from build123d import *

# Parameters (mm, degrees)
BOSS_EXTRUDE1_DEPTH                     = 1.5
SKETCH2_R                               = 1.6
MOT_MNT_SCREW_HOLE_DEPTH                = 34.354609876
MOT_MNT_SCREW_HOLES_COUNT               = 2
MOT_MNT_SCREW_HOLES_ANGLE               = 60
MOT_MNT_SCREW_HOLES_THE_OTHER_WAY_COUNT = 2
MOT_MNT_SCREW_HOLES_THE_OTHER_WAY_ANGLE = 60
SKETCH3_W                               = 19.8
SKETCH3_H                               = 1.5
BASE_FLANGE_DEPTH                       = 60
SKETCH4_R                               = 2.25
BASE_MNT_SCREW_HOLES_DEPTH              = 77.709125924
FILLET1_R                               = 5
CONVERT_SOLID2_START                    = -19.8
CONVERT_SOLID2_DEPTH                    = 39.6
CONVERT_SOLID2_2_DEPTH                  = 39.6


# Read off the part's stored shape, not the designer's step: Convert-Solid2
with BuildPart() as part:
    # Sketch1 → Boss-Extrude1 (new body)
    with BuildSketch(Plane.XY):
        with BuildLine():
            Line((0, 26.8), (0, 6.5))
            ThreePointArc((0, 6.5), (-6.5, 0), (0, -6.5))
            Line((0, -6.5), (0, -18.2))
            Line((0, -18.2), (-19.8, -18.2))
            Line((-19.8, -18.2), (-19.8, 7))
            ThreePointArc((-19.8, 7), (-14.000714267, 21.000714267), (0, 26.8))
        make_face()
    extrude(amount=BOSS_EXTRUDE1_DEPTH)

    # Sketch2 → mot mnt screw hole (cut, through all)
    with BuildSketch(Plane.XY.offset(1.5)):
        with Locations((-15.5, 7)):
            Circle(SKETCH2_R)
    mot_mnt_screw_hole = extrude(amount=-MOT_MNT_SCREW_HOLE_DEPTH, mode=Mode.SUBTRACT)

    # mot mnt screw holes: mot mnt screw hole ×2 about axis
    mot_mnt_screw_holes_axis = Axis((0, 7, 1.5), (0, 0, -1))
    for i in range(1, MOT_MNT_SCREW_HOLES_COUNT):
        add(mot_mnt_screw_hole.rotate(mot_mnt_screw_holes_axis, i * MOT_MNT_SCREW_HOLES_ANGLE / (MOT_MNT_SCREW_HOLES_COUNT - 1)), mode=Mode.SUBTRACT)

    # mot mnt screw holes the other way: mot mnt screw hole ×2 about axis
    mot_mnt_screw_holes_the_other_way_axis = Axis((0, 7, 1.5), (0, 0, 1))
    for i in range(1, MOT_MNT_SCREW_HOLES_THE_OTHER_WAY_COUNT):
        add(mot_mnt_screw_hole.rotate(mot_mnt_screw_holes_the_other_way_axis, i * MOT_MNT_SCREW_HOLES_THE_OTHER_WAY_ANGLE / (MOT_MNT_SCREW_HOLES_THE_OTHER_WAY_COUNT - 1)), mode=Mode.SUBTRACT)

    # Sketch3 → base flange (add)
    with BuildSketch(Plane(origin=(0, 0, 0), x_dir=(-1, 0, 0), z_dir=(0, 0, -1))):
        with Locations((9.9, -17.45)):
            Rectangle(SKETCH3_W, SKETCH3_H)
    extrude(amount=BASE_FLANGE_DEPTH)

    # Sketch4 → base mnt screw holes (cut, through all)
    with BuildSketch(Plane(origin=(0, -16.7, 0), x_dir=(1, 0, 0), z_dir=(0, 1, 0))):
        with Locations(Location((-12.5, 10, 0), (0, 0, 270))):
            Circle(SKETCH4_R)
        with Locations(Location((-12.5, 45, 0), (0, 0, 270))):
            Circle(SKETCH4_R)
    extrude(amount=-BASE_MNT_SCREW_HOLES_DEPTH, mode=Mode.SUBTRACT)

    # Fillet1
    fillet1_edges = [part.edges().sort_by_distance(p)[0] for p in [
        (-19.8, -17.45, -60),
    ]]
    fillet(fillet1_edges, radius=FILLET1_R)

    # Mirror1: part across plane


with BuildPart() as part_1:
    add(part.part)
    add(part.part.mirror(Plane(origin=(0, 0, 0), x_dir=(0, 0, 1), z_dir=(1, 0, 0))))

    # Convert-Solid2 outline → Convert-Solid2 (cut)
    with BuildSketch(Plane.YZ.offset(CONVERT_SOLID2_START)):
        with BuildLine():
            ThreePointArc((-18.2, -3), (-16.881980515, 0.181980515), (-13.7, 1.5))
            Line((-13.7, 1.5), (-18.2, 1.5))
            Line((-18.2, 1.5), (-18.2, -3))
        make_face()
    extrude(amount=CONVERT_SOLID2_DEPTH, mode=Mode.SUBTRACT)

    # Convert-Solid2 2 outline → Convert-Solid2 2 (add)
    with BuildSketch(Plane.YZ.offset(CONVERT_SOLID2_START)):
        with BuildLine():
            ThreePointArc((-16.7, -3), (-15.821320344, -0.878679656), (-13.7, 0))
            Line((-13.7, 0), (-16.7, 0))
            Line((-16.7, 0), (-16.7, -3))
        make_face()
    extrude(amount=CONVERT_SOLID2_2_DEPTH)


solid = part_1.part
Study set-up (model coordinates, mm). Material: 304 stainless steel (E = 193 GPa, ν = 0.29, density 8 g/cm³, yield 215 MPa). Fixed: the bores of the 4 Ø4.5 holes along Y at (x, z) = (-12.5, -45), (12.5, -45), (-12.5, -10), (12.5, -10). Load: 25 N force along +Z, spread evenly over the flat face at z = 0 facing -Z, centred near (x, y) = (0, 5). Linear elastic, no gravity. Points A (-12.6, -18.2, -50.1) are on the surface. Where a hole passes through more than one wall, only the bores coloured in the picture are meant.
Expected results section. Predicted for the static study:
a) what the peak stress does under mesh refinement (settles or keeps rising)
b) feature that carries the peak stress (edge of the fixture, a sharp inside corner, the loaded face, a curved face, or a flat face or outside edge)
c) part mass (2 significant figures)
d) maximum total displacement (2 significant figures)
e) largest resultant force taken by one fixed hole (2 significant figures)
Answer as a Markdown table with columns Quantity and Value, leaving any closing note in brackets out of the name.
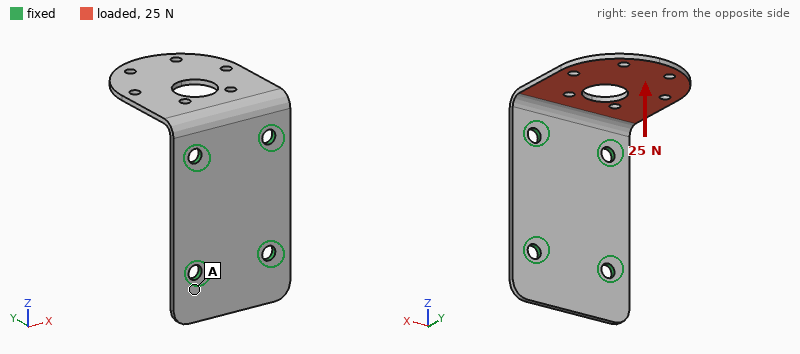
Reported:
| Quantity | Value |
|---|---|
| what the peak stress does under mesh refinement | keeps rising |
| feature that carries the peak stress | edge of the fixture |
| part mass | 44 g |
| maximum total displacement | 0.24 mm |
| largest resultant force taken by one fixed hole | 10 N |
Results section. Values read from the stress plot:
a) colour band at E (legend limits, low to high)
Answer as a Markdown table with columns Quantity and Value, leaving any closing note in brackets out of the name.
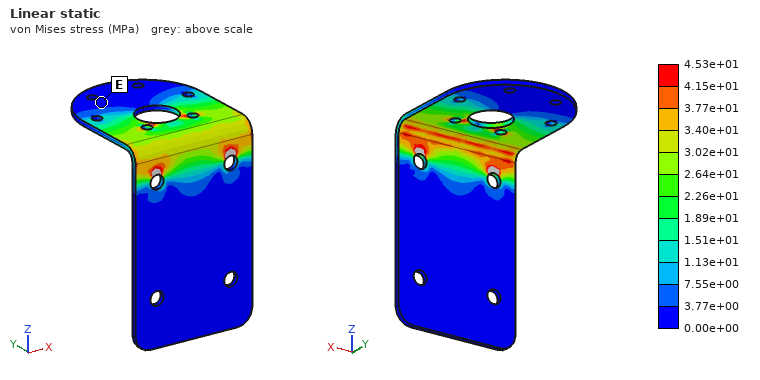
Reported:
| Quantity | Value |
|---|---|
| colour band at E | 0.00e+00 to 3.77e+00 MPa |
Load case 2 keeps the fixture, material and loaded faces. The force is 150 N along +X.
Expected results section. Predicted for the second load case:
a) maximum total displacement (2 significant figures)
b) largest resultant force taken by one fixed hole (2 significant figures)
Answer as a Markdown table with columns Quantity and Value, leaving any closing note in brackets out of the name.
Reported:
| Quantity | Value |
|---|---|
| maximum total displacement | 91 µm |
| largest resultant force taken by one fixed hole | 150 N |
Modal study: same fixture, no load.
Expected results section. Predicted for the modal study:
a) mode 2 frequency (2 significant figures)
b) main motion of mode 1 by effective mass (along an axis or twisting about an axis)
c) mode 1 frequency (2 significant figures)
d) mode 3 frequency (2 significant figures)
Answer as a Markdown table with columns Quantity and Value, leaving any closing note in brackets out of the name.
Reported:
| Quantity | Value |
|---|---|
| mode 2 frequency | 1600 Hz |
| main motion of mode 1 by effective mass | along Z |
| mode 1 frequency | 540 Hz |
| mode 3 frequency | 2500 Hz |
